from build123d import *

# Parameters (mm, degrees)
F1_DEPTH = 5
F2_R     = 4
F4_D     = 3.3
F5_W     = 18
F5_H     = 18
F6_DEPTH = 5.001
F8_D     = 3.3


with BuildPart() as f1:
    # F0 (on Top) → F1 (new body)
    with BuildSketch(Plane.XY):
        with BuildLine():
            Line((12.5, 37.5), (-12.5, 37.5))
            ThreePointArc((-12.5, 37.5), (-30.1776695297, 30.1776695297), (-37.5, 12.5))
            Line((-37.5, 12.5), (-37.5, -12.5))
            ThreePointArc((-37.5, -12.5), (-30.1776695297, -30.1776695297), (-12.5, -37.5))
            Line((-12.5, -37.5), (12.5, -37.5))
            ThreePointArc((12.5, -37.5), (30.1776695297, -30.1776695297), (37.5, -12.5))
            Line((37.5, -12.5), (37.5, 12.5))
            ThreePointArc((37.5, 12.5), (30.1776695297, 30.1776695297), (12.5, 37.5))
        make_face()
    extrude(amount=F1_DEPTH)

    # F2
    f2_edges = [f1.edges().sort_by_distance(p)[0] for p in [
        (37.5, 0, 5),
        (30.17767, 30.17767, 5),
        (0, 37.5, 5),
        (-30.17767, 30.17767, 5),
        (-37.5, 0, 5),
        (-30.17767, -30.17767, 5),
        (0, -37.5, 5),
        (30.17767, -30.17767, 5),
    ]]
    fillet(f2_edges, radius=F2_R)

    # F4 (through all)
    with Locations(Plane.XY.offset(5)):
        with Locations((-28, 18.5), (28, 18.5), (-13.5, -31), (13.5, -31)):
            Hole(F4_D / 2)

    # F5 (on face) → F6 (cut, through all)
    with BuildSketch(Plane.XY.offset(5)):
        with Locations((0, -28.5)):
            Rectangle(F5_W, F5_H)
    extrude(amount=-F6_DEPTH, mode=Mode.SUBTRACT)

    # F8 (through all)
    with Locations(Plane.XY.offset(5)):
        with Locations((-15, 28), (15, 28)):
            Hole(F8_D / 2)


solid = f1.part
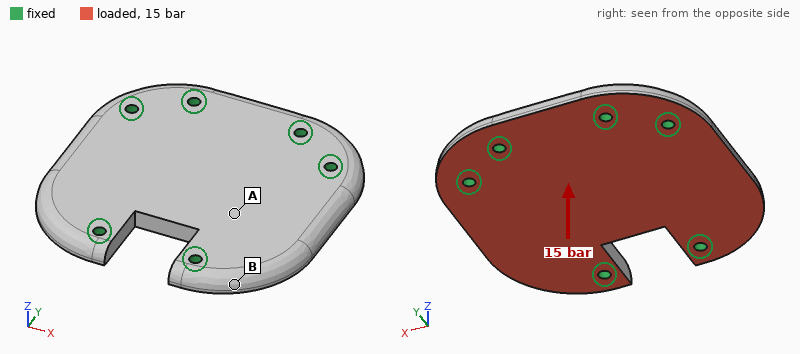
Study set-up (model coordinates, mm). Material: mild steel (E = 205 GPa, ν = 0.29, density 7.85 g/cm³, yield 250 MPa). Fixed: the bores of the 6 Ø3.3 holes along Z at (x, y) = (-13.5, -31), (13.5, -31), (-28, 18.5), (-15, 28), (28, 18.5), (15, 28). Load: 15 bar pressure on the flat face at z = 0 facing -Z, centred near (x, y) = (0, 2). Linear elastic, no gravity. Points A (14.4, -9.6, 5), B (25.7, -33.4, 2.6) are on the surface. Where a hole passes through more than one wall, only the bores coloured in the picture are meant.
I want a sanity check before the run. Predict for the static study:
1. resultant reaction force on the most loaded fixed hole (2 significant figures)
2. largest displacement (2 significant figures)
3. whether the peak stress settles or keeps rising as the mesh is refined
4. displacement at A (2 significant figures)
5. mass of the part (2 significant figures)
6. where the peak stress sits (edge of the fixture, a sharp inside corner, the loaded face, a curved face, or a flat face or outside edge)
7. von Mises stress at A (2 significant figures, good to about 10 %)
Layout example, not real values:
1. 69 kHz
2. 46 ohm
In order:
1. 1.4 kN
2. 33 µm
3. keeps rising
4. 21 µm
5. 180 g
6. edge of the fixture
7. 49 MPa
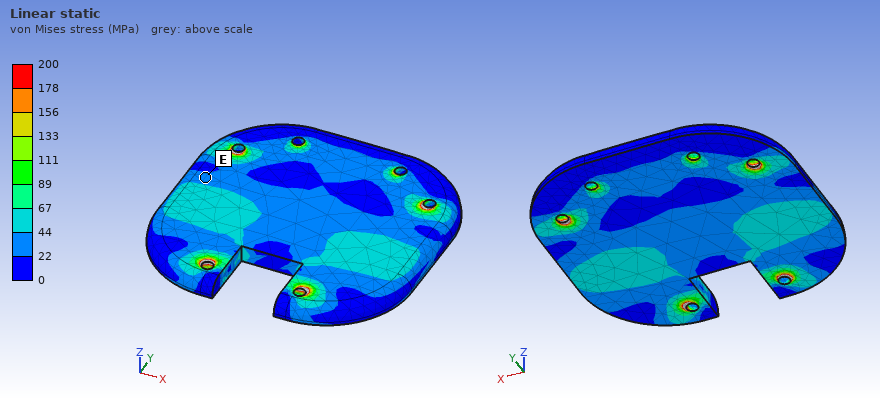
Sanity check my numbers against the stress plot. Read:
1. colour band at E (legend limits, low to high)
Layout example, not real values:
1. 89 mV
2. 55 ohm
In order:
1. 22 to 44 MPa
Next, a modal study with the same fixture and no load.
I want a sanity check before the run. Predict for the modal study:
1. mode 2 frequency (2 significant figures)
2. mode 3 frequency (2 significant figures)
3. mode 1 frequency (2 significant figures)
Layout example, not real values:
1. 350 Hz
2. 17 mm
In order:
1. 7300 Hz
2. 8900 Hz
3. 7000 Hz
